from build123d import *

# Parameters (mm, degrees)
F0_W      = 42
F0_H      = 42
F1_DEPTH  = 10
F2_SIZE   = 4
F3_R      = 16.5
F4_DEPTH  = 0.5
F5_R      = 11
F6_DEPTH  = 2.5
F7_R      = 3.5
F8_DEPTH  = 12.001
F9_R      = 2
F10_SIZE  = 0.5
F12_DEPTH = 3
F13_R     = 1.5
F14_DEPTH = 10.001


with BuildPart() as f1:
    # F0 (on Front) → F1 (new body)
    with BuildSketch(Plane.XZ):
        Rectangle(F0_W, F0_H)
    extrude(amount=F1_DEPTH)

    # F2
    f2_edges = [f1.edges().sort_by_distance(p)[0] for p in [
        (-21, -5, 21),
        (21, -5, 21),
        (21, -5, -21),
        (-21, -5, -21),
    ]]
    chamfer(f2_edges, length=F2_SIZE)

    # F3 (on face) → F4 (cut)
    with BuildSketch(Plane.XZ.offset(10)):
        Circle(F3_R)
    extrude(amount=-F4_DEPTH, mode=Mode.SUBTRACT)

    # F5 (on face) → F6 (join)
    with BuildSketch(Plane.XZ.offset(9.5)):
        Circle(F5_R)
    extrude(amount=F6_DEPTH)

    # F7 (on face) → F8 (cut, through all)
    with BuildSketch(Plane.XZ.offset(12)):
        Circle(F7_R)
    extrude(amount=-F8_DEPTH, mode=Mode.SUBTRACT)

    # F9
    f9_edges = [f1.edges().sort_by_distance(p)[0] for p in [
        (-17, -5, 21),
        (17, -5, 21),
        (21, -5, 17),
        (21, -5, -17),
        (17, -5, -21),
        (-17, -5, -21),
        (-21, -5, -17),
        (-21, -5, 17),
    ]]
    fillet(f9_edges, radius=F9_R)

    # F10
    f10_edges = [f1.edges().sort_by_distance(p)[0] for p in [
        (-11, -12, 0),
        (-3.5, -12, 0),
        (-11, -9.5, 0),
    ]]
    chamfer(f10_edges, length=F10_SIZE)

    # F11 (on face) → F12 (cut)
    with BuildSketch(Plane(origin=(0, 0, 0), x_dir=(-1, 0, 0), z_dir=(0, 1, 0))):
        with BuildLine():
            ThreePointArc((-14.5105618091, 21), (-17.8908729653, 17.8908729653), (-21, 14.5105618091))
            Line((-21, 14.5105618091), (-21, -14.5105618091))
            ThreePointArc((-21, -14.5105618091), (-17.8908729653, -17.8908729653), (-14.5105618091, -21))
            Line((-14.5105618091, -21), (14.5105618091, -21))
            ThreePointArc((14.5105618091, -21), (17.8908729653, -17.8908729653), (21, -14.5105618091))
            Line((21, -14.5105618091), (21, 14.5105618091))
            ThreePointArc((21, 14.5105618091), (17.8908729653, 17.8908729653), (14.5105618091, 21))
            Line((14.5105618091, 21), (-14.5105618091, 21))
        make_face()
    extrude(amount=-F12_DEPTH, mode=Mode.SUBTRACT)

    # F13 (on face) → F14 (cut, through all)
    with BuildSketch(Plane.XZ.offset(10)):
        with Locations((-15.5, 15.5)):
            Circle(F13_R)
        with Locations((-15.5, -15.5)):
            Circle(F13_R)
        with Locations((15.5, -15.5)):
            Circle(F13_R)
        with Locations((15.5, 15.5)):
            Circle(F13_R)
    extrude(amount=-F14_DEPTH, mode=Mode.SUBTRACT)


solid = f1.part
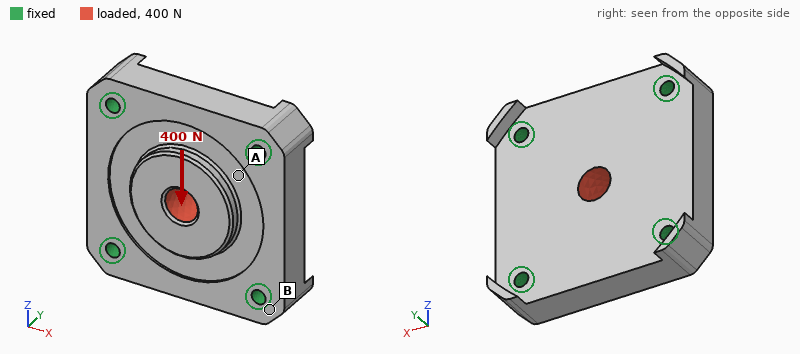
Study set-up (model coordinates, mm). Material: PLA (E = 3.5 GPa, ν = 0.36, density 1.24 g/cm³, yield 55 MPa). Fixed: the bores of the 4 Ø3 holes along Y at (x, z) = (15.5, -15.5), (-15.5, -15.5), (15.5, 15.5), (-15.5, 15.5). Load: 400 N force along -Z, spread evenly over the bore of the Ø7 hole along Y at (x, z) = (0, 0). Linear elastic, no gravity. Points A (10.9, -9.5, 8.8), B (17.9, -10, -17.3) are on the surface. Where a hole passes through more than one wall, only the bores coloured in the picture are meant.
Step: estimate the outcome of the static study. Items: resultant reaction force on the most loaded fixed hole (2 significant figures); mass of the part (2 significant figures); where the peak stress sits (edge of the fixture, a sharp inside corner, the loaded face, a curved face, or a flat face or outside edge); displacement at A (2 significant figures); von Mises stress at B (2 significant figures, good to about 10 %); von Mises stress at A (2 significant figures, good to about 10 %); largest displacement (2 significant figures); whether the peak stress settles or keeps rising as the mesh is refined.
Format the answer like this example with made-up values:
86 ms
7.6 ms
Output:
110 N
15 g
edge of the fixture
4.3 µm
0.64 MPa
2.0 MPa
12 µm
keeps rising
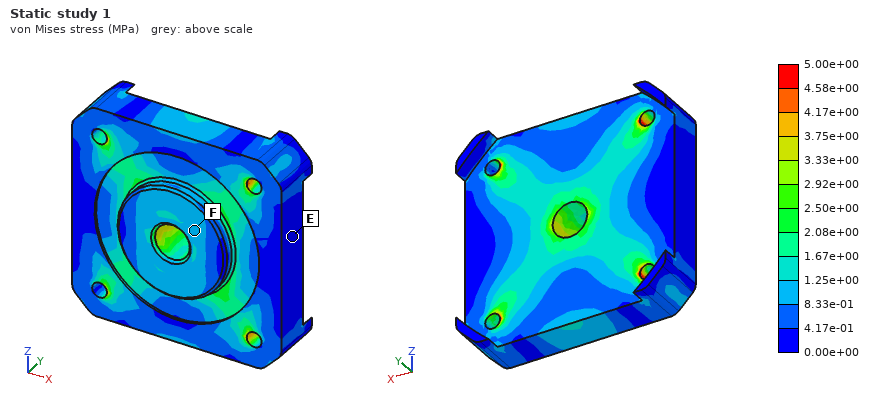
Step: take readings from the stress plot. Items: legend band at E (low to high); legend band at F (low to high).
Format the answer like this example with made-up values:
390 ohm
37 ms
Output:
0.00e+00 to 4.17e-01 MPa
8.33e-01 to 1.25e+00 MPa
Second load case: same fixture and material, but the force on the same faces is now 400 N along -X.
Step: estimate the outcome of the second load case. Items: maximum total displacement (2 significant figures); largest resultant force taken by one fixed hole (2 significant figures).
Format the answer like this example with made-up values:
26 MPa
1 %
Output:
12 µm
110 N
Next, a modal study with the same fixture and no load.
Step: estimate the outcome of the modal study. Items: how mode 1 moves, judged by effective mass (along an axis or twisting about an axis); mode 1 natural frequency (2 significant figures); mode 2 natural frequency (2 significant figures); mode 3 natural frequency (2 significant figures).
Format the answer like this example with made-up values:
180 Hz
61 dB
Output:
along Y
6900 Hz
10000 Hz
10000 Hz
